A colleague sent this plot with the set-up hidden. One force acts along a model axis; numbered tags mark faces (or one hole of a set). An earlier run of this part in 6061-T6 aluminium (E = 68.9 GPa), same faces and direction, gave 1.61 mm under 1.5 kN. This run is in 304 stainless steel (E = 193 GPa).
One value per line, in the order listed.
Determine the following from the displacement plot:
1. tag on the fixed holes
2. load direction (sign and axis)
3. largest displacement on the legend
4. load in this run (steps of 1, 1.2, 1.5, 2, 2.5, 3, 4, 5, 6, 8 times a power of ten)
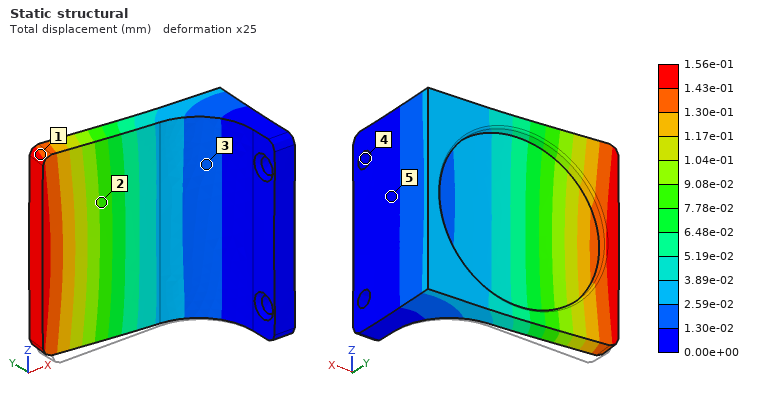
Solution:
4
+Y
1.56e-01 mm
400 N
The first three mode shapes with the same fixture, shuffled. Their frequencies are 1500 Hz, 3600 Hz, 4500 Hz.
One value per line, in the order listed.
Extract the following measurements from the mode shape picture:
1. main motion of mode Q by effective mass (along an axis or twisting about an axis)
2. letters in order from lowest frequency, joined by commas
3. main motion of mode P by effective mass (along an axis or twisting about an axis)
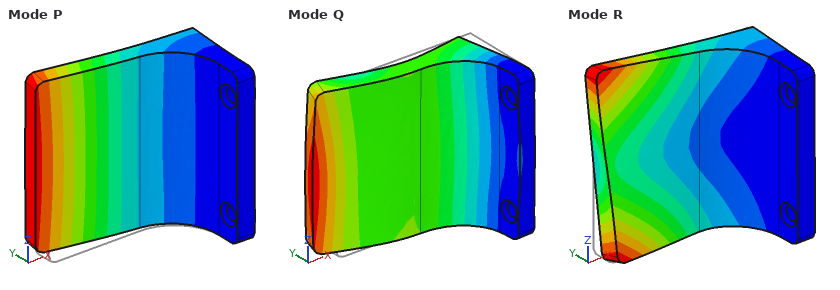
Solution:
along X
P, R, Q
along Y
